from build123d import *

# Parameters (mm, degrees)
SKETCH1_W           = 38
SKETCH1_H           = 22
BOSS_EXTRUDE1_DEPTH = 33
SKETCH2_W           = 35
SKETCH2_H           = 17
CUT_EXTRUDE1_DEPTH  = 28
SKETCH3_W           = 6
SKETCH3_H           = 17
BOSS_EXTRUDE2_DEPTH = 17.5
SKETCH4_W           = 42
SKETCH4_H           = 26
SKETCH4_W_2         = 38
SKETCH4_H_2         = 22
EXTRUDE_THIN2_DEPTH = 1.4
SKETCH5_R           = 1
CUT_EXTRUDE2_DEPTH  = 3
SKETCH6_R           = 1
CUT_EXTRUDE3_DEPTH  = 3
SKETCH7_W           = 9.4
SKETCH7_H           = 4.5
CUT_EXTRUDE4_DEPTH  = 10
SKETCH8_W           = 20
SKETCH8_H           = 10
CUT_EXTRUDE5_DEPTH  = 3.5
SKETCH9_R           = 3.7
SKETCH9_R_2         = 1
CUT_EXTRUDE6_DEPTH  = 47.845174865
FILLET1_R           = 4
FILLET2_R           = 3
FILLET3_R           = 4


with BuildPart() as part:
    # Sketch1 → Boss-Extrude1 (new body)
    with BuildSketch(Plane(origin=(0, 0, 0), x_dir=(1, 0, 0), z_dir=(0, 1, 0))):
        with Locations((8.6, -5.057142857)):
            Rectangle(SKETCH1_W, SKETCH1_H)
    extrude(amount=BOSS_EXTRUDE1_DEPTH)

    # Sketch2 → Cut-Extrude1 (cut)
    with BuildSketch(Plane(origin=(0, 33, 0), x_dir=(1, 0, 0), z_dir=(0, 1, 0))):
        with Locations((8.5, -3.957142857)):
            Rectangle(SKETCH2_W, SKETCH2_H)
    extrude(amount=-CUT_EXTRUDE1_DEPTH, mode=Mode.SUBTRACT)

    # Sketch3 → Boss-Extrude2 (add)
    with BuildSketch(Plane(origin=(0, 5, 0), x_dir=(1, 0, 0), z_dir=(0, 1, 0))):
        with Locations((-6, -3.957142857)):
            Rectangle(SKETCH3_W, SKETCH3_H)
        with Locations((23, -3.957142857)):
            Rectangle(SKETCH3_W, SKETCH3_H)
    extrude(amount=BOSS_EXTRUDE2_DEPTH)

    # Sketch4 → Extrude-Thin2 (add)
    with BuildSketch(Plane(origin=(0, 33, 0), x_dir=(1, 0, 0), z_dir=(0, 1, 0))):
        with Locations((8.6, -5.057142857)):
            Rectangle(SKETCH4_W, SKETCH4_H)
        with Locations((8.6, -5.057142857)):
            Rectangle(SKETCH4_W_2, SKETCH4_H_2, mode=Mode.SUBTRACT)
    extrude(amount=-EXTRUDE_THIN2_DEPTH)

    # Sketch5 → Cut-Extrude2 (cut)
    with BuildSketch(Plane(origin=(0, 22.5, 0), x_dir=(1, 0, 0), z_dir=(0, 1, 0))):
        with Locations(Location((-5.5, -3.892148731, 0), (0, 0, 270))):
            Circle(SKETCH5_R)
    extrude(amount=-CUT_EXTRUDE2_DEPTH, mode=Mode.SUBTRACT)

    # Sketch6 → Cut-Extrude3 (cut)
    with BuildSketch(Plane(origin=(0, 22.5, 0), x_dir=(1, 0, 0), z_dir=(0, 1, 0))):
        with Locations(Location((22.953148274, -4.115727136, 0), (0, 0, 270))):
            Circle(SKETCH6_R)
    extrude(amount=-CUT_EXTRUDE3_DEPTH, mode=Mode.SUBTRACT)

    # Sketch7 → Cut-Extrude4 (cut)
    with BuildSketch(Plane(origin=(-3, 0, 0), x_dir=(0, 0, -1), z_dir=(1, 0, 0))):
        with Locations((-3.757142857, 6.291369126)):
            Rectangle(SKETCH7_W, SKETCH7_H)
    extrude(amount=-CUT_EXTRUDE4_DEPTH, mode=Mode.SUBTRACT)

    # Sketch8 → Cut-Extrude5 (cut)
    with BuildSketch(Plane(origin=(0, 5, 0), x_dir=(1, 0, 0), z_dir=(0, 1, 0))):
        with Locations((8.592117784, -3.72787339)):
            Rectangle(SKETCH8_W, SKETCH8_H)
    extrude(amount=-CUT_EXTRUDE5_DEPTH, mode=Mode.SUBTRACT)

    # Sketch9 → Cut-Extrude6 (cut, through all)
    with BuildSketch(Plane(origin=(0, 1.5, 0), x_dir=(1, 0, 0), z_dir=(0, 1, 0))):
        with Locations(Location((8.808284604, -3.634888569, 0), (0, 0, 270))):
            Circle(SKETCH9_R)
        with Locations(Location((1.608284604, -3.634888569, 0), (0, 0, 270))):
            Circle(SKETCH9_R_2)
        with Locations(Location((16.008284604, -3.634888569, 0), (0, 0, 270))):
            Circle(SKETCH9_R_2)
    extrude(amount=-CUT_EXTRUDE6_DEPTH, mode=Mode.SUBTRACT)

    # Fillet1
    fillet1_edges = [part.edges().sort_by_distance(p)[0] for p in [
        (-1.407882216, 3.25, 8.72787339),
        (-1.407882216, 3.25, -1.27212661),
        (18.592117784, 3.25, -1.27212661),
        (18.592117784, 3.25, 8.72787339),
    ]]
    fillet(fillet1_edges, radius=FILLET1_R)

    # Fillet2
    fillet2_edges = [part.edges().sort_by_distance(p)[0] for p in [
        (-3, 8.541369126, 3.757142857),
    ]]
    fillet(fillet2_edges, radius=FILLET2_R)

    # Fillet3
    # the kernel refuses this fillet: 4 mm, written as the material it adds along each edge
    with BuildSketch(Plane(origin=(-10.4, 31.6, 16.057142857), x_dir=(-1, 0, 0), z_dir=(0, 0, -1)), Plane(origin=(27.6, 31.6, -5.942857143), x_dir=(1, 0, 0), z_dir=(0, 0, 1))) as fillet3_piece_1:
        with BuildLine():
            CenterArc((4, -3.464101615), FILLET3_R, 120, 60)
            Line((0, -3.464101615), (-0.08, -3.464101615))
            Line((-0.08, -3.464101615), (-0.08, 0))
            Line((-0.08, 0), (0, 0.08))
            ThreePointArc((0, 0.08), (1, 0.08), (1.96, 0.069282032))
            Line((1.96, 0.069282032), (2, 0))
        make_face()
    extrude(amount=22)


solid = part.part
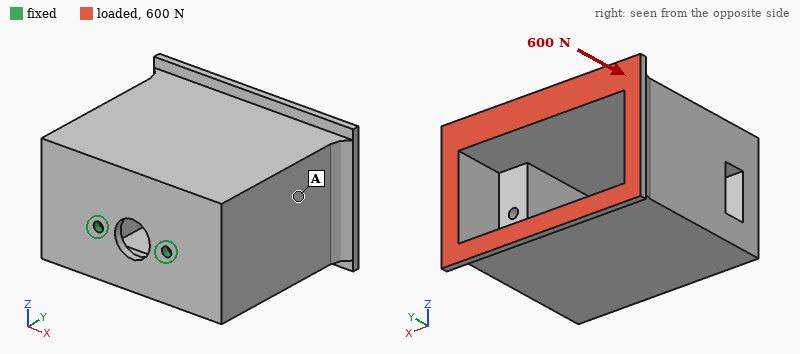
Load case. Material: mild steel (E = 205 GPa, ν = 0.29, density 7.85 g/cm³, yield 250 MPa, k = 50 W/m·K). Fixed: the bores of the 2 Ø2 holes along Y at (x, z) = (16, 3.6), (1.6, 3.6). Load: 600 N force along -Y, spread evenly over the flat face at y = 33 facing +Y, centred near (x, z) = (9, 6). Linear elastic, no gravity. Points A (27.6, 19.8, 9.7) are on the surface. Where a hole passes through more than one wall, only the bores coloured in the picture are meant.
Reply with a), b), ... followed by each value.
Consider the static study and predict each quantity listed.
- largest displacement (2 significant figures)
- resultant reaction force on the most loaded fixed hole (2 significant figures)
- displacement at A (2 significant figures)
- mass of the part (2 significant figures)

a) 50 µm
b) 320 N
c) 28 µm
d) 110 g
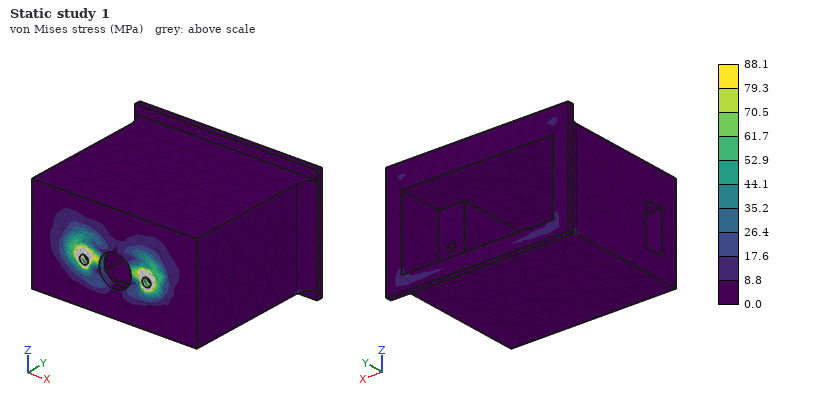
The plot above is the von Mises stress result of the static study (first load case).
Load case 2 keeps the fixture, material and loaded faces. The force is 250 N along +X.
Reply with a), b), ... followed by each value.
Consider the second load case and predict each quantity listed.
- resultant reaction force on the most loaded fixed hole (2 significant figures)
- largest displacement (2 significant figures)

a) 490 N
b) 25 µm
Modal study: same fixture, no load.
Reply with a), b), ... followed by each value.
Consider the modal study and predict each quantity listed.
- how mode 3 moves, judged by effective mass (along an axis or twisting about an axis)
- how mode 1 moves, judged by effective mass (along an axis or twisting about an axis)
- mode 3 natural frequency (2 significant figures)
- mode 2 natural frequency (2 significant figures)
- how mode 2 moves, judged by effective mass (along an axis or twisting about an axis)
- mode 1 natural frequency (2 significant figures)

a) twisting about Y
b) along Z
c) 5800 Hz
d) 2600 Hz
e) along X
f) 910 Hz
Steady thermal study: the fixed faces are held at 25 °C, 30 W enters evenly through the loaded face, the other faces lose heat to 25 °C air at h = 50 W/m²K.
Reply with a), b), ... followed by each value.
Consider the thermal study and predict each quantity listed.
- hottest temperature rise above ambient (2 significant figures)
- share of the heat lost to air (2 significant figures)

a) 74 K
b) 58 %
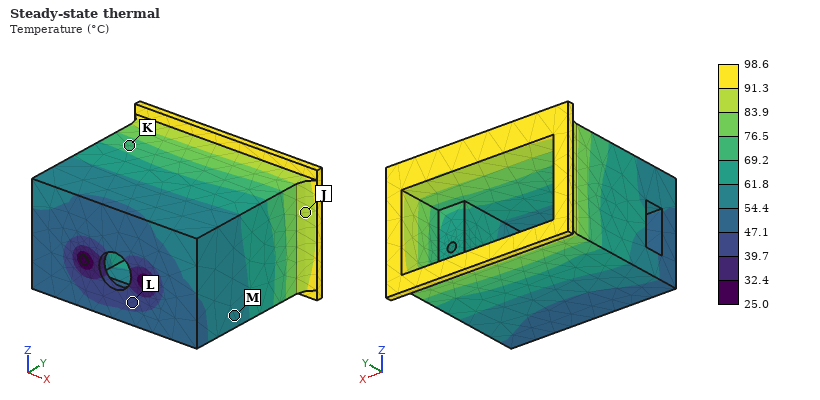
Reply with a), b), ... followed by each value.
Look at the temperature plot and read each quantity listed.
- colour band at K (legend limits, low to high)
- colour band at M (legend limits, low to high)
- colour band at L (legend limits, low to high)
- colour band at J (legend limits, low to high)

a) 69.2 to 76.5 °C
b) 54.4 to 61.8 °C
c) 39.7 to 47.1 °C
d) 83.9 to 91.3 °C
